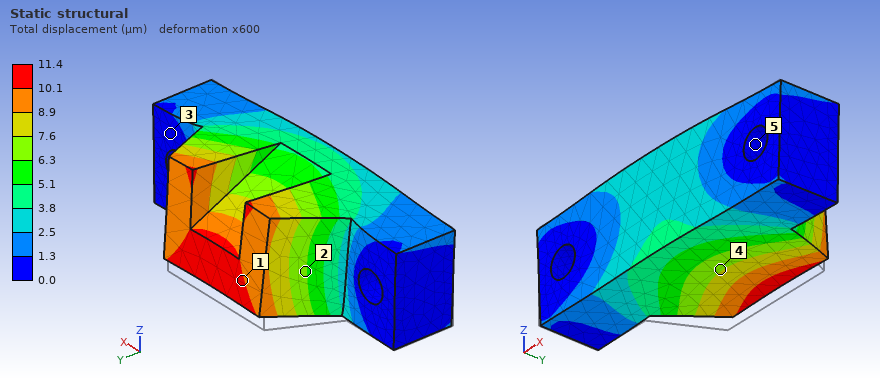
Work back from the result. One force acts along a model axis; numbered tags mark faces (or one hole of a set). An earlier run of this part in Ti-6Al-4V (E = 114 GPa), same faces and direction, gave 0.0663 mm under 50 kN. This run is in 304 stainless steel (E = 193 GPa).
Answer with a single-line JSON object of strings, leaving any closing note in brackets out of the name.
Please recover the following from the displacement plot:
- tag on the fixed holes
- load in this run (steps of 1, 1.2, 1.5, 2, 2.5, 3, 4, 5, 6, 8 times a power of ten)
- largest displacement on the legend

{"tag on the fixed holes": "5", "load in this run": "15 kN", "largest displacement on the legend": "11.4 µm"}
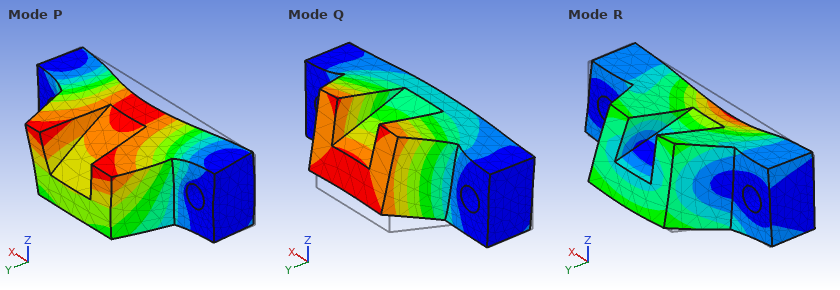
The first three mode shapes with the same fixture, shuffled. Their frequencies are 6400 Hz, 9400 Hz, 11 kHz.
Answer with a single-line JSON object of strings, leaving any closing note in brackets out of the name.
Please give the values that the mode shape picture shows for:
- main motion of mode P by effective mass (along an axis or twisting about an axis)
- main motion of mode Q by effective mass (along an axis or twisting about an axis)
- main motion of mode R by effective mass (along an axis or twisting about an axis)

{"main motion of mode P by effective mass": "along Y", "main motion of mode Q by effective mass": "along Z", "main motion of mode R by effective mass": "along Z"}
